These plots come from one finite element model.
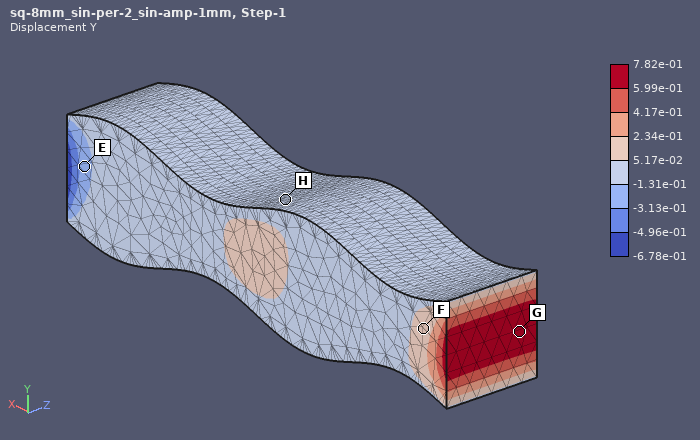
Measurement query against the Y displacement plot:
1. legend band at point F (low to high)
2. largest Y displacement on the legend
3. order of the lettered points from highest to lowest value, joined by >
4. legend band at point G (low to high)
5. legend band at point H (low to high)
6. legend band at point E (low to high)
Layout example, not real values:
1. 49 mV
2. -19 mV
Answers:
1. 5.17e-02 to 2.34e-01
2. 7.82e-01
3. G > F > H > E
4. 5.99e-01 to 7.82e-01
5. -1.31e-01 to 5.17e-02
6. -3.13e-01 to -1.31e-01
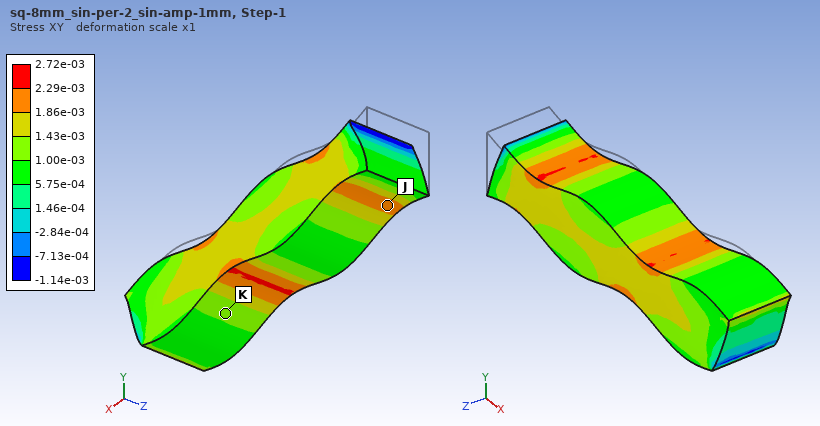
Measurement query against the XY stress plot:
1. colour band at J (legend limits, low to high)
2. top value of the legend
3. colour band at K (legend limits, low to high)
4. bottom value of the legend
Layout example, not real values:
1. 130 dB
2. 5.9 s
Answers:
1. 1.86e-03 to 2.29e-03
2. 2.72e-03
3. 1.00e-03 to 1.43e-03
4. -1.14e-03
